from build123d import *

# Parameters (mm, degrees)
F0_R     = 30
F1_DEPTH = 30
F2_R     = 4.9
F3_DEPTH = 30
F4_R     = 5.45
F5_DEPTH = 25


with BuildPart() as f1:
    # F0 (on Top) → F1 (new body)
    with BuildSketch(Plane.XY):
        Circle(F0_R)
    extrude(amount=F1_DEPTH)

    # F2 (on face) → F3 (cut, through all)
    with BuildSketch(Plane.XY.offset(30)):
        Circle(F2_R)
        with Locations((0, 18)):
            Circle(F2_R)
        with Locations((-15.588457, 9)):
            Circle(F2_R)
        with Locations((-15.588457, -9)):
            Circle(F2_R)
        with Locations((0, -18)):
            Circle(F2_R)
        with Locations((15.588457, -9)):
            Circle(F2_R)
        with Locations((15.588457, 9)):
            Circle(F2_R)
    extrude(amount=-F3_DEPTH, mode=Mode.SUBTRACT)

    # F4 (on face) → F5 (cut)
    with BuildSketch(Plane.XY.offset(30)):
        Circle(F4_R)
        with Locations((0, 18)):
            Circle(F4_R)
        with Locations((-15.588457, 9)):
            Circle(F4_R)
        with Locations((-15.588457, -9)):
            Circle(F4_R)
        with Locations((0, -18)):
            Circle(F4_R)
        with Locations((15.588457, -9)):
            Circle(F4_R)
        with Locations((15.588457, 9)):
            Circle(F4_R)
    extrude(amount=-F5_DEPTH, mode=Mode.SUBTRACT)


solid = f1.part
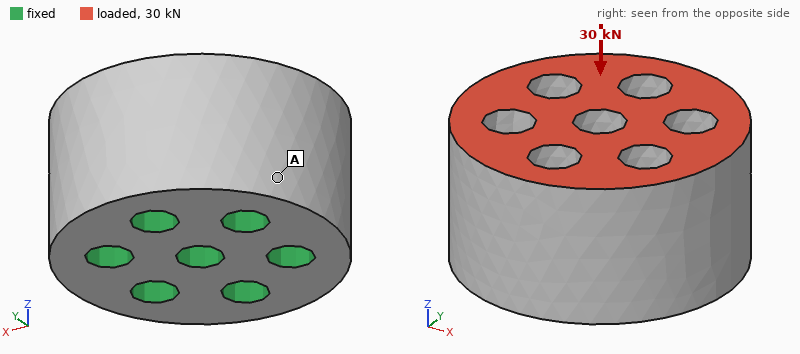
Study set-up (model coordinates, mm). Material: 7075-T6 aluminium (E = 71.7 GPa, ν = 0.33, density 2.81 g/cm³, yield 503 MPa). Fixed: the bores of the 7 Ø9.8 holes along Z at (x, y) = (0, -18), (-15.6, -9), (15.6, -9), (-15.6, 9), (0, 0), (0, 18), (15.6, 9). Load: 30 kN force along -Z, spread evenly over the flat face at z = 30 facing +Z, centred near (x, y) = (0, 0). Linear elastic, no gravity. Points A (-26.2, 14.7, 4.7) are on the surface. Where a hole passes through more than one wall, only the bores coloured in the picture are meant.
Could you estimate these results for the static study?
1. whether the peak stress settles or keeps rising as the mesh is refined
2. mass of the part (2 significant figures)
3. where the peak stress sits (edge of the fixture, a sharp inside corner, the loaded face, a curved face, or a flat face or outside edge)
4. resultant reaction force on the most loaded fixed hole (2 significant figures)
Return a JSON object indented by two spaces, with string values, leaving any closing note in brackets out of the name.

{
  "whether the peak stress settles or keeps rising as the mesh is refined": "keeps rising",
  "mass of the part": "190 g",
  "where the peak stress sits": "edge of the fixture",
  "resultant reaction force on the most loaded fixed hole": "4.5 kN"
}
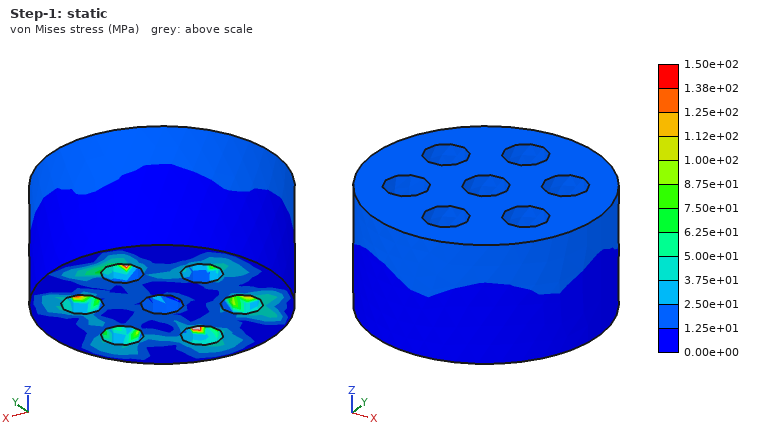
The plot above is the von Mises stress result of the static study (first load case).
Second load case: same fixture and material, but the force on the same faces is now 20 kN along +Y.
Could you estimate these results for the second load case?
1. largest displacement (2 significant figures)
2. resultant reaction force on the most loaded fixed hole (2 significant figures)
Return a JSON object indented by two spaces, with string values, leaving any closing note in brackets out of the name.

{
  "largest displacement": "41 µm",
  "resultant reaction force on the most loaded fixed hole": "8.9 kN"
}
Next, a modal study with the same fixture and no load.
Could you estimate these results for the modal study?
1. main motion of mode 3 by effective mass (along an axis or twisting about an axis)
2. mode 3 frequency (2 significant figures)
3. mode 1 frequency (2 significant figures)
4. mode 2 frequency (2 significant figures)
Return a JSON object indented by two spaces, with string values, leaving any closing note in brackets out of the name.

{
  "main motion of mode 3 by effective mass": "twisting about Z",
  "mode 3 frequency": "23 kHz",
  "mode 1 frequency": "15 kHz",
  "mode 2 frequency": "15 kHz"
}
